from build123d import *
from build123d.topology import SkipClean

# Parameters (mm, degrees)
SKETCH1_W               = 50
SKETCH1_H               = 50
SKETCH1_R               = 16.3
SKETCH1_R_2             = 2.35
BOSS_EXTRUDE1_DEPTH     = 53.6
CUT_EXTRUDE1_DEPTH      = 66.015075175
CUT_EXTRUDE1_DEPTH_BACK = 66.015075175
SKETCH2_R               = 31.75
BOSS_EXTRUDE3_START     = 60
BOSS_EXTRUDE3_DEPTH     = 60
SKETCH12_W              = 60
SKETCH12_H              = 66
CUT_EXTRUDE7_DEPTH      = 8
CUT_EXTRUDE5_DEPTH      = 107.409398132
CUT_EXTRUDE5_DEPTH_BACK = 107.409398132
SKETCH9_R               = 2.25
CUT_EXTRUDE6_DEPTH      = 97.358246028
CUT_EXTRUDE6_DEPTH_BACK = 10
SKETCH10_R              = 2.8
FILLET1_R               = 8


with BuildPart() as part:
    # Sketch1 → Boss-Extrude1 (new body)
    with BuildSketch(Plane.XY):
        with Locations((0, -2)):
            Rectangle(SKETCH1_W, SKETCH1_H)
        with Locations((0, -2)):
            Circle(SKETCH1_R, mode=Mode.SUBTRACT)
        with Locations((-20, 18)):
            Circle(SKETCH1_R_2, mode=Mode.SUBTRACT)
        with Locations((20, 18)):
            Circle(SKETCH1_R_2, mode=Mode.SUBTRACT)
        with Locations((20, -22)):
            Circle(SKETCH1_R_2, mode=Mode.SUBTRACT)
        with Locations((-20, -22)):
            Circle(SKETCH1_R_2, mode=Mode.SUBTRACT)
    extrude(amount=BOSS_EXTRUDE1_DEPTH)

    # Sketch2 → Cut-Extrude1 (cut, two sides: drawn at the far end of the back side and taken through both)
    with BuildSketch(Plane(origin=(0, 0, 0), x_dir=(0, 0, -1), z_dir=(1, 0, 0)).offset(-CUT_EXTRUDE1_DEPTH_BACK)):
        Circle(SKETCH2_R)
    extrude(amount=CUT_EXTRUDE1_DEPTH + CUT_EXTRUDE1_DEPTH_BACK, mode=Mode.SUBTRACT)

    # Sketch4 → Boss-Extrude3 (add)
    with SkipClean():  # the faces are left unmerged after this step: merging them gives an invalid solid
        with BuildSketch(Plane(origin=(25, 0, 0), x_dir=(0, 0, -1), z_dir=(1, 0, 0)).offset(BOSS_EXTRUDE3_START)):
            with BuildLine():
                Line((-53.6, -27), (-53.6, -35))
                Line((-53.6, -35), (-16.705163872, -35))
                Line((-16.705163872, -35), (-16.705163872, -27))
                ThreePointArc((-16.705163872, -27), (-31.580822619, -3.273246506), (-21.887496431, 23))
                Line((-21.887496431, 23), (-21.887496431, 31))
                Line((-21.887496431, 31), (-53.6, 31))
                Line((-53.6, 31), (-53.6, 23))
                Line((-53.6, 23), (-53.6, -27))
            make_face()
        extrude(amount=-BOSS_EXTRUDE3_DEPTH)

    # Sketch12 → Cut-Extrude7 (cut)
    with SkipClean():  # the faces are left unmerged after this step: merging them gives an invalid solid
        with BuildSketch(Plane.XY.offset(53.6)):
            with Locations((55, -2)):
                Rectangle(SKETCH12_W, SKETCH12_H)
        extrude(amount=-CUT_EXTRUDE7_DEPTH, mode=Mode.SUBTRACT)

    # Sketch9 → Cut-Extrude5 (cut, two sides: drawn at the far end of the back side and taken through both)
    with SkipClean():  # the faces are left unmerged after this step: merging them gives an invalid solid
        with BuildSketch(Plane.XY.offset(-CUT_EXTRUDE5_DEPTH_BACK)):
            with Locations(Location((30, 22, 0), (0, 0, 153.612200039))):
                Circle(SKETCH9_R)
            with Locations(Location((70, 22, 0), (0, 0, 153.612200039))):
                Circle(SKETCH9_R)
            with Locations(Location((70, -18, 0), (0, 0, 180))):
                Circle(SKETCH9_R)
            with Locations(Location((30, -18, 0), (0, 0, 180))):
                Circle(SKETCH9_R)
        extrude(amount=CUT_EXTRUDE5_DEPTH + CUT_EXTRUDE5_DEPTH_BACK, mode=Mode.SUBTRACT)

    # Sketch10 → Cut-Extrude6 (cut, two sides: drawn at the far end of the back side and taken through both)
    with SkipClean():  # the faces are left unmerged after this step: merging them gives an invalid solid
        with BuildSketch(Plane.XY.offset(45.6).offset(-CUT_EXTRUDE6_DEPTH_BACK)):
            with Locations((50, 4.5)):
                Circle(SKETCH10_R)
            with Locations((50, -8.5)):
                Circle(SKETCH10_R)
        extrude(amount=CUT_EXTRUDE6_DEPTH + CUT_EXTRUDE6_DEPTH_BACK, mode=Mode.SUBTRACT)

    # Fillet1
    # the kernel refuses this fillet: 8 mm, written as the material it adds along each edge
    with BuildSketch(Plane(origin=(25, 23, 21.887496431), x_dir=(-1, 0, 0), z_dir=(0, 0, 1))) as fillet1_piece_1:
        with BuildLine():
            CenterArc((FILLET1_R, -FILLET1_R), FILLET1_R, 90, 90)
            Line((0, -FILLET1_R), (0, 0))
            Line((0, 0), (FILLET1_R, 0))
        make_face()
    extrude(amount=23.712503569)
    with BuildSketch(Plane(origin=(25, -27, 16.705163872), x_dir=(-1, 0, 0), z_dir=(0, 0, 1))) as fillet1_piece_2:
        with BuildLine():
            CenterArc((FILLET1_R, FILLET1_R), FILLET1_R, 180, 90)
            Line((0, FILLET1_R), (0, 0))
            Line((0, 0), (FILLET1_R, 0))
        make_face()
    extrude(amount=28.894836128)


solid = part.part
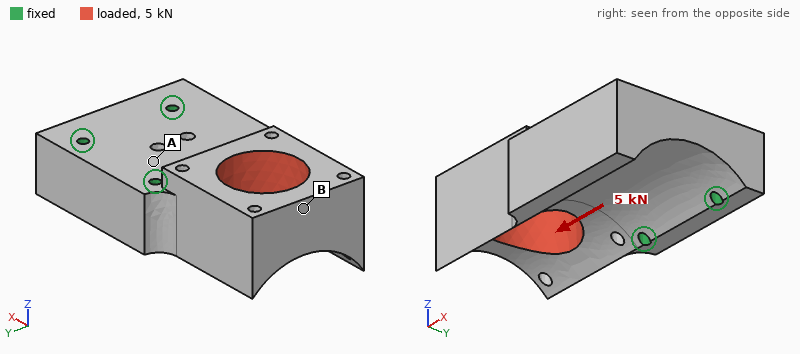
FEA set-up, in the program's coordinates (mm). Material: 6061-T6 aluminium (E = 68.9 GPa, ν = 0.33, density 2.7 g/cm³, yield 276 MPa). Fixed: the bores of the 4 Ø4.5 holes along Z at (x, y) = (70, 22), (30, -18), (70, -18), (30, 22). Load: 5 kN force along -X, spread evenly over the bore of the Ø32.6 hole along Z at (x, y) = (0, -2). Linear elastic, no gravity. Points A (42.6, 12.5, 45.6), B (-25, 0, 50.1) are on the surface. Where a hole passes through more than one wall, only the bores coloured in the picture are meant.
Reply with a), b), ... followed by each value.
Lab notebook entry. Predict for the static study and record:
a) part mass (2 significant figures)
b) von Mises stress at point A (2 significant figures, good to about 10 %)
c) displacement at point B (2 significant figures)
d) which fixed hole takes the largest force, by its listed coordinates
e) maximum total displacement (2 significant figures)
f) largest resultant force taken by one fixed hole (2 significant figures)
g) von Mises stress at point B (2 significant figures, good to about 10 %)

a) 320 g
b) 3.5 MPa
c) 19 µm
d) (30, -18)
e) 19 µm
f) 2.4 kN
g) 9.8 MPa
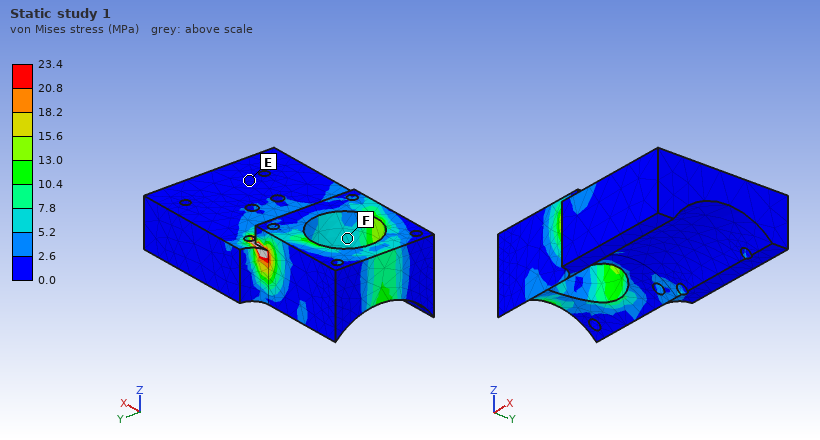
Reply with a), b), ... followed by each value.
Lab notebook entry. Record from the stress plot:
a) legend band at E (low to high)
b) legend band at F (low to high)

a) 0.0 to 2.6 MPa
b) 5.2 to 7.8 MPa
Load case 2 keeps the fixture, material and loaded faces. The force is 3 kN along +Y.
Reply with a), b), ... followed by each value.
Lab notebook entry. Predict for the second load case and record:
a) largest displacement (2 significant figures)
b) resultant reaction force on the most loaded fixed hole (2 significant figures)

a) 28 µm
b) 2.3 kN
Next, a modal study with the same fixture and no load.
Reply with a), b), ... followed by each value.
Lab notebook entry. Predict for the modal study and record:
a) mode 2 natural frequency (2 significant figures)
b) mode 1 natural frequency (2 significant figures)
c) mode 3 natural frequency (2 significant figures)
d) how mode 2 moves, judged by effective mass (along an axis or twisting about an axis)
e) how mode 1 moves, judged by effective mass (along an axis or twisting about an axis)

a) 5500 Hz
b) 4400 Hz
c) 7400 Hz
d) along Y
e) along Z
